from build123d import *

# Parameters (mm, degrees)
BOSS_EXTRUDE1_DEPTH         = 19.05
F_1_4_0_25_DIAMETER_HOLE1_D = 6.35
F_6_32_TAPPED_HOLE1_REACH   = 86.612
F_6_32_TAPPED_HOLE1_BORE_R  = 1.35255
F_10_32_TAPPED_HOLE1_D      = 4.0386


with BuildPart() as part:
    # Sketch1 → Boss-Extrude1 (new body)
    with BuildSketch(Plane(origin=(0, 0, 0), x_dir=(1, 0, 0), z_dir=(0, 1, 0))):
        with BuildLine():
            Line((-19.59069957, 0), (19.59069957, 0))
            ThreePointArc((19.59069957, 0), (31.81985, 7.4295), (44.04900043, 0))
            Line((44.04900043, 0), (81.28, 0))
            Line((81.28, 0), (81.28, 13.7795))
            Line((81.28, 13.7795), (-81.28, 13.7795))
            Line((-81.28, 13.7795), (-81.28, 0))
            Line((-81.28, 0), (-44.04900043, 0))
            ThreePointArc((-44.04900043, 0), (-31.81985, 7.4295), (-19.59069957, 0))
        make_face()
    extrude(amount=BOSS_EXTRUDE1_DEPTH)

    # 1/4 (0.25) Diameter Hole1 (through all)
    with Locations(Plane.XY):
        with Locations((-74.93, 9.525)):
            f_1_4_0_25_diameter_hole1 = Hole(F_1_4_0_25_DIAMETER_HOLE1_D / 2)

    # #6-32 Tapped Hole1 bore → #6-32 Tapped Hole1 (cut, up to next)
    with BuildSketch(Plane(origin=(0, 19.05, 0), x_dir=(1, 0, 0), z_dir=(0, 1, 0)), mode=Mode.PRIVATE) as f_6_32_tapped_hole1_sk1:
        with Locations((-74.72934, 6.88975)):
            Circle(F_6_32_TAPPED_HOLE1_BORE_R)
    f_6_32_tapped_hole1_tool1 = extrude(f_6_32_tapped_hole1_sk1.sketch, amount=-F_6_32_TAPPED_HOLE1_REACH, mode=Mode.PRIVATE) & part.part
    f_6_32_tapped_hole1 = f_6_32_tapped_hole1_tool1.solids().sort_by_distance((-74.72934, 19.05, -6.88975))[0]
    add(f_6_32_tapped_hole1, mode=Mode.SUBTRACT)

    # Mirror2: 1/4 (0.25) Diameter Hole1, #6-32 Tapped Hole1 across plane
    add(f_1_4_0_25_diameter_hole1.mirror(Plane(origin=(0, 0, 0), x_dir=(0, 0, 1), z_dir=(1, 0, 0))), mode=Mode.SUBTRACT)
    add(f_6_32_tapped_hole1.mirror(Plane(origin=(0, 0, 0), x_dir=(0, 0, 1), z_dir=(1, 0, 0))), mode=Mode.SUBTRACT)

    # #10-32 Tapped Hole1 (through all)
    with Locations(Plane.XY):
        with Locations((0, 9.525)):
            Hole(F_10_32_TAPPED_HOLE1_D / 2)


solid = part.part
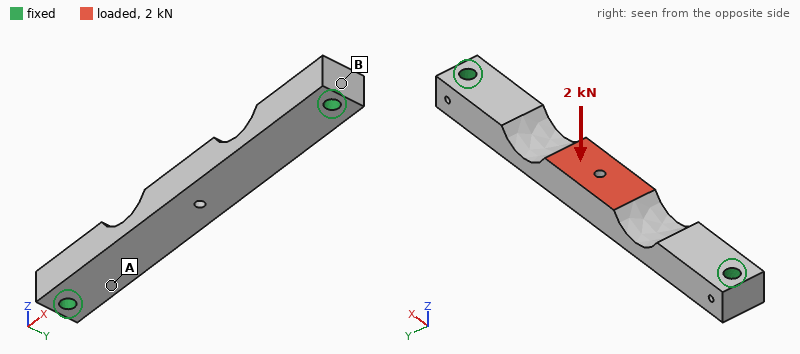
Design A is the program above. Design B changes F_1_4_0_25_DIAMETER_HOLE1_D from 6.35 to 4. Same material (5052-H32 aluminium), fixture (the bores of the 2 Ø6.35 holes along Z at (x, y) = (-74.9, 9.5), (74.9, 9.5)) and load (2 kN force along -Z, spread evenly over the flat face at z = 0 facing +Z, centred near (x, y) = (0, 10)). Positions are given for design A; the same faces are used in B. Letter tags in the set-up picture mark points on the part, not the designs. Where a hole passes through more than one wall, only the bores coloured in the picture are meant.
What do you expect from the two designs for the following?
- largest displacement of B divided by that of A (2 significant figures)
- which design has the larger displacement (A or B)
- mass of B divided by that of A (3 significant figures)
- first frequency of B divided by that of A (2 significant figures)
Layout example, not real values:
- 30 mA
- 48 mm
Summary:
- 1.1
- B
- 1.01
- 0.94
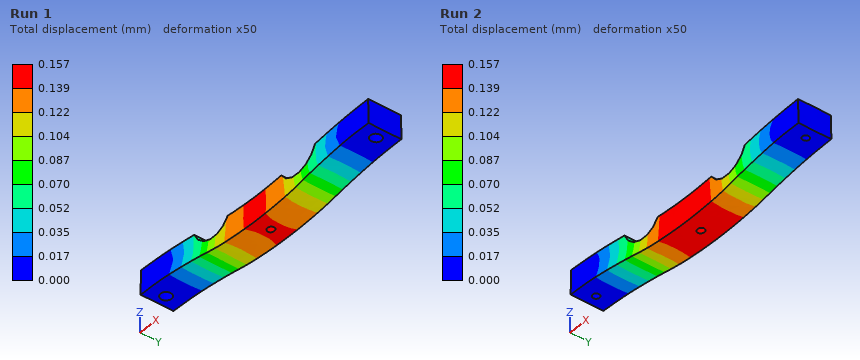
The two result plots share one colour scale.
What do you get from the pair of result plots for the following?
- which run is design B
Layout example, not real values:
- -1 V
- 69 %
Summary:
- Run 2
